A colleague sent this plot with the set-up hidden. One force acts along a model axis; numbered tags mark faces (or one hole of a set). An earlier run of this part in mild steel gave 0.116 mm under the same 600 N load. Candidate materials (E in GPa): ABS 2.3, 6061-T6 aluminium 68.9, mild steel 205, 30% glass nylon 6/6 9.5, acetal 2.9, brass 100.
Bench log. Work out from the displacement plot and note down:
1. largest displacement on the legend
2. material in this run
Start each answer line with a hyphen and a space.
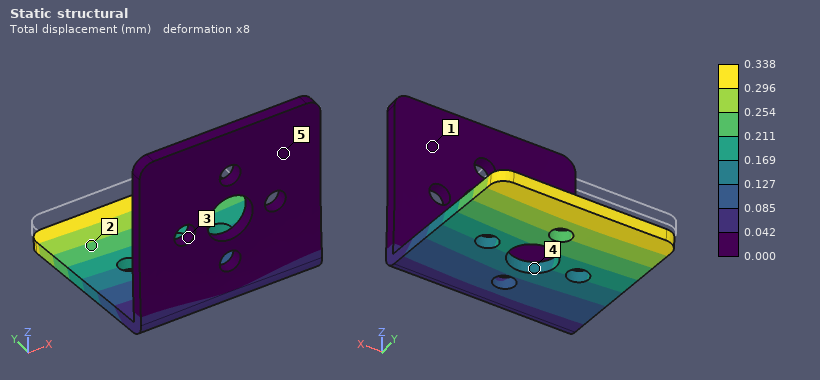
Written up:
- 0.338 mm
- 6061-T6 aluminium
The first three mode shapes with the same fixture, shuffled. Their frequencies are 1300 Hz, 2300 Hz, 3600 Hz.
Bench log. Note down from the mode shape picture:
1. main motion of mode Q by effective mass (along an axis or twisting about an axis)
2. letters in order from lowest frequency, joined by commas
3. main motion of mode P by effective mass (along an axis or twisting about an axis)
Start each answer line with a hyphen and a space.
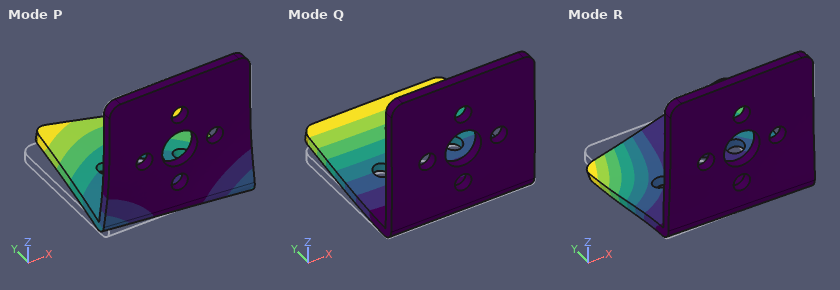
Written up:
- along Z
- Q, P, R
- along X
